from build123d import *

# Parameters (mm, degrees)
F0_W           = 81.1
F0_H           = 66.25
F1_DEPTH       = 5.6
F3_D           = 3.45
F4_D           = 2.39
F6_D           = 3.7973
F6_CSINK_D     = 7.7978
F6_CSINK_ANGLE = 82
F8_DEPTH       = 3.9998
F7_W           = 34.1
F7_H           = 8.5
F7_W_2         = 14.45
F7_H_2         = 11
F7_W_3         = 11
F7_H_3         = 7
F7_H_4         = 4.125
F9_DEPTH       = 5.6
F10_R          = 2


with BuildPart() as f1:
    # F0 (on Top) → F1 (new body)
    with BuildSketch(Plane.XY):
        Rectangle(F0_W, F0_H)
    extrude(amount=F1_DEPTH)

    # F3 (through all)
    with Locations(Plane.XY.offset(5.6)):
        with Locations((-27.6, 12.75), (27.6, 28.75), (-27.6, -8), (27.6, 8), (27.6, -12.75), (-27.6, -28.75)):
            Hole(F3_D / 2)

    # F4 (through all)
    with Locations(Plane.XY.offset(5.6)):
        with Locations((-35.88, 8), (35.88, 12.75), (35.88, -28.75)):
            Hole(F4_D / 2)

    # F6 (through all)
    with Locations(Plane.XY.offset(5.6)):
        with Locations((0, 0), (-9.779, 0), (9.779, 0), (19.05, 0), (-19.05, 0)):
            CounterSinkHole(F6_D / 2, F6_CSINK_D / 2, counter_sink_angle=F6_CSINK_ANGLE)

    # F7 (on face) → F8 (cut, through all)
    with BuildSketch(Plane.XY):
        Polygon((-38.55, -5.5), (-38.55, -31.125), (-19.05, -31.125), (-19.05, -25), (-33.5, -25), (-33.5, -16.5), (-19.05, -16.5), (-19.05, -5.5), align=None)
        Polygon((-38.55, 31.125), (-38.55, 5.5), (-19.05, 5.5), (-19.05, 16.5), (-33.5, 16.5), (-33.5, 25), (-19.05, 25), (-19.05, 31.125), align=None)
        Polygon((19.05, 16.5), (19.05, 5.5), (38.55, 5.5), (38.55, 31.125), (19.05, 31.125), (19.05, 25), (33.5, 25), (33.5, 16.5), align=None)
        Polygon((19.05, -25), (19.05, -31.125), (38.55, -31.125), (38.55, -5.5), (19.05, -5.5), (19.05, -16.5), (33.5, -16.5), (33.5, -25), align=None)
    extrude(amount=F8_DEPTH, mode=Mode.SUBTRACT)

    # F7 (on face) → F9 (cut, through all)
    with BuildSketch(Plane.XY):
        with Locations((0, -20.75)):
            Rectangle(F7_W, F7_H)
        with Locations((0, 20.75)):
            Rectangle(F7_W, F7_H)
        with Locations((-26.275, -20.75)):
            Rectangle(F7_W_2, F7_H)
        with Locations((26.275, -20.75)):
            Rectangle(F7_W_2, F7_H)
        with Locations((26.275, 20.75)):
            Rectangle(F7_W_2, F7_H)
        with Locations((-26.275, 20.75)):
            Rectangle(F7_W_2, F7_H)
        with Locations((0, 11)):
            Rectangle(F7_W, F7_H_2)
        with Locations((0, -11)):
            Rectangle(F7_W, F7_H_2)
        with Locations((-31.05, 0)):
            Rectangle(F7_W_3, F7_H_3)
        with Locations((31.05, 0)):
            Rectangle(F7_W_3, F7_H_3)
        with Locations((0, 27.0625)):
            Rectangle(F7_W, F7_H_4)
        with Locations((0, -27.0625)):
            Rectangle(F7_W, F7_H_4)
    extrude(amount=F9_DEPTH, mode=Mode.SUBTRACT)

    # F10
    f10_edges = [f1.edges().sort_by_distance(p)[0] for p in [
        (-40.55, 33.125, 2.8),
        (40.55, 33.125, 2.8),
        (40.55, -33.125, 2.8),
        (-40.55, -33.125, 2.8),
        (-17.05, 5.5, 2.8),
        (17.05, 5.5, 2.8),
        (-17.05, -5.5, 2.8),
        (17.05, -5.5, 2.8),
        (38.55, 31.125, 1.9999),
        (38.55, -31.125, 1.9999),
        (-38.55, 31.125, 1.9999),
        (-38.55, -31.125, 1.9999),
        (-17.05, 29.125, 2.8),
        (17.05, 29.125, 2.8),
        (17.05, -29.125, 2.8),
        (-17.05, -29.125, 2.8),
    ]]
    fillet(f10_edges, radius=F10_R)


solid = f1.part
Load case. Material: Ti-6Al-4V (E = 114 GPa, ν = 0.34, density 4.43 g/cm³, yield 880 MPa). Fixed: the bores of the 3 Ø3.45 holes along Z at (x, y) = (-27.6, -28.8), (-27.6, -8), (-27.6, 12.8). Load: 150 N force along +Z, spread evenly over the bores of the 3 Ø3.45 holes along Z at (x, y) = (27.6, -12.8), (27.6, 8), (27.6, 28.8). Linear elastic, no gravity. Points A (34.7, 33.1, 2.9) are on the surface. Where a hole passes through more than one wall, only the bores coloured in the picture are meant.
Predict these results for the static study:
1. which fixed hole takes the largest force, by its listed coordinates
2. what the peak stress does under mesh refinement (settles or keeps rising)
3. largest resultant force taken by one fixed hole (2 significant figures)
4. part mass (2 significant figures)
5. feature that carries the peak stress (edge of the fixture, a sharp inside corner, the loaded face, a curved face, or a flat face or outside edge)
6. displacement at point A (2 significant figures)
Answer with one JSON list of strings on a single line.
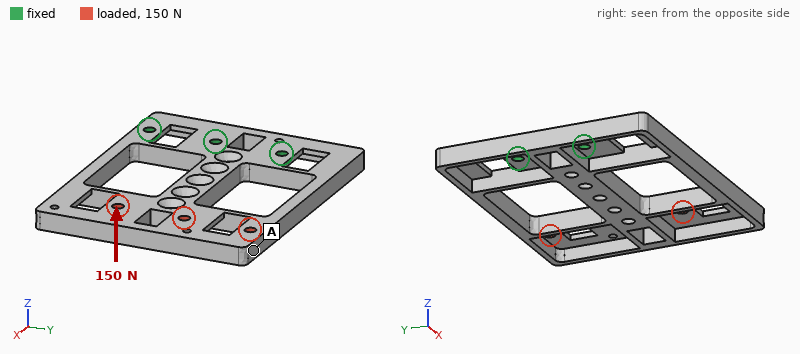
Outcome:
["(-27.6, -8)", "keeps rising", "260 N", "48 g", "edge of the fixture", "1.00 mm"]
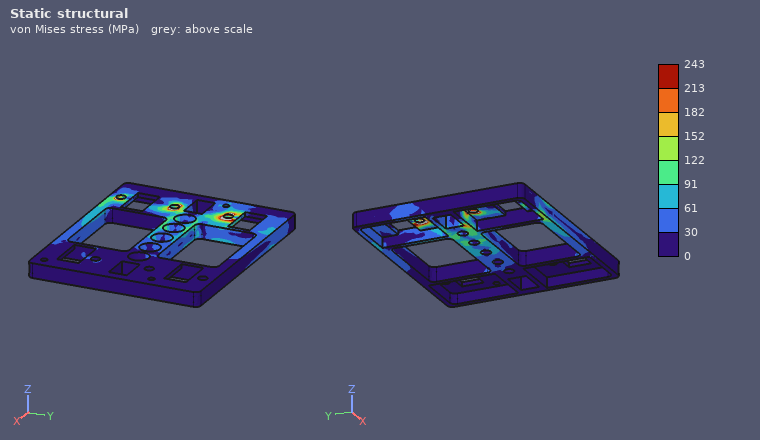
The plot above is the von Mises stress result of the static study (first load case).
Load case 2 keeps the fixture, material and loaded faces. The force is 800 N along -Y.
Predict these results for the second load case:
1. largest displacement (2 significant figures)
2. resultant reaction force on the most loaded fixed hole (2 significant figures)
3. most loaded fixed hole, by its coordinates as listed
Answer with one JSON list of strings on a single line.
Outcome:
["0.28 mm", "1.6 kN", "(-27.6, 12.8)"]
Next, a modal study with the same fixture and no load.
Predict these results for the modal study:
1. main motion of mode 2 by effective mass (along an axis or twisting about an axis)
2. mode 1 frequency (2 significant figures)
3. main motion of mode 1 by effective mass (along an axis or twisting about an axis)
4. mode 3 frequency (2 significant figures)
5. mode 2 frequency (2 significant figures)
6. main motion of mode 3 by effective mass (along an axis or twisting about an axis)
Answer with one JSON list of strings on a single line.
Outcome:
["twisting about X", "510 Hz", "along Z", "2400 Hz", "1100 Hz", "along Y"]
